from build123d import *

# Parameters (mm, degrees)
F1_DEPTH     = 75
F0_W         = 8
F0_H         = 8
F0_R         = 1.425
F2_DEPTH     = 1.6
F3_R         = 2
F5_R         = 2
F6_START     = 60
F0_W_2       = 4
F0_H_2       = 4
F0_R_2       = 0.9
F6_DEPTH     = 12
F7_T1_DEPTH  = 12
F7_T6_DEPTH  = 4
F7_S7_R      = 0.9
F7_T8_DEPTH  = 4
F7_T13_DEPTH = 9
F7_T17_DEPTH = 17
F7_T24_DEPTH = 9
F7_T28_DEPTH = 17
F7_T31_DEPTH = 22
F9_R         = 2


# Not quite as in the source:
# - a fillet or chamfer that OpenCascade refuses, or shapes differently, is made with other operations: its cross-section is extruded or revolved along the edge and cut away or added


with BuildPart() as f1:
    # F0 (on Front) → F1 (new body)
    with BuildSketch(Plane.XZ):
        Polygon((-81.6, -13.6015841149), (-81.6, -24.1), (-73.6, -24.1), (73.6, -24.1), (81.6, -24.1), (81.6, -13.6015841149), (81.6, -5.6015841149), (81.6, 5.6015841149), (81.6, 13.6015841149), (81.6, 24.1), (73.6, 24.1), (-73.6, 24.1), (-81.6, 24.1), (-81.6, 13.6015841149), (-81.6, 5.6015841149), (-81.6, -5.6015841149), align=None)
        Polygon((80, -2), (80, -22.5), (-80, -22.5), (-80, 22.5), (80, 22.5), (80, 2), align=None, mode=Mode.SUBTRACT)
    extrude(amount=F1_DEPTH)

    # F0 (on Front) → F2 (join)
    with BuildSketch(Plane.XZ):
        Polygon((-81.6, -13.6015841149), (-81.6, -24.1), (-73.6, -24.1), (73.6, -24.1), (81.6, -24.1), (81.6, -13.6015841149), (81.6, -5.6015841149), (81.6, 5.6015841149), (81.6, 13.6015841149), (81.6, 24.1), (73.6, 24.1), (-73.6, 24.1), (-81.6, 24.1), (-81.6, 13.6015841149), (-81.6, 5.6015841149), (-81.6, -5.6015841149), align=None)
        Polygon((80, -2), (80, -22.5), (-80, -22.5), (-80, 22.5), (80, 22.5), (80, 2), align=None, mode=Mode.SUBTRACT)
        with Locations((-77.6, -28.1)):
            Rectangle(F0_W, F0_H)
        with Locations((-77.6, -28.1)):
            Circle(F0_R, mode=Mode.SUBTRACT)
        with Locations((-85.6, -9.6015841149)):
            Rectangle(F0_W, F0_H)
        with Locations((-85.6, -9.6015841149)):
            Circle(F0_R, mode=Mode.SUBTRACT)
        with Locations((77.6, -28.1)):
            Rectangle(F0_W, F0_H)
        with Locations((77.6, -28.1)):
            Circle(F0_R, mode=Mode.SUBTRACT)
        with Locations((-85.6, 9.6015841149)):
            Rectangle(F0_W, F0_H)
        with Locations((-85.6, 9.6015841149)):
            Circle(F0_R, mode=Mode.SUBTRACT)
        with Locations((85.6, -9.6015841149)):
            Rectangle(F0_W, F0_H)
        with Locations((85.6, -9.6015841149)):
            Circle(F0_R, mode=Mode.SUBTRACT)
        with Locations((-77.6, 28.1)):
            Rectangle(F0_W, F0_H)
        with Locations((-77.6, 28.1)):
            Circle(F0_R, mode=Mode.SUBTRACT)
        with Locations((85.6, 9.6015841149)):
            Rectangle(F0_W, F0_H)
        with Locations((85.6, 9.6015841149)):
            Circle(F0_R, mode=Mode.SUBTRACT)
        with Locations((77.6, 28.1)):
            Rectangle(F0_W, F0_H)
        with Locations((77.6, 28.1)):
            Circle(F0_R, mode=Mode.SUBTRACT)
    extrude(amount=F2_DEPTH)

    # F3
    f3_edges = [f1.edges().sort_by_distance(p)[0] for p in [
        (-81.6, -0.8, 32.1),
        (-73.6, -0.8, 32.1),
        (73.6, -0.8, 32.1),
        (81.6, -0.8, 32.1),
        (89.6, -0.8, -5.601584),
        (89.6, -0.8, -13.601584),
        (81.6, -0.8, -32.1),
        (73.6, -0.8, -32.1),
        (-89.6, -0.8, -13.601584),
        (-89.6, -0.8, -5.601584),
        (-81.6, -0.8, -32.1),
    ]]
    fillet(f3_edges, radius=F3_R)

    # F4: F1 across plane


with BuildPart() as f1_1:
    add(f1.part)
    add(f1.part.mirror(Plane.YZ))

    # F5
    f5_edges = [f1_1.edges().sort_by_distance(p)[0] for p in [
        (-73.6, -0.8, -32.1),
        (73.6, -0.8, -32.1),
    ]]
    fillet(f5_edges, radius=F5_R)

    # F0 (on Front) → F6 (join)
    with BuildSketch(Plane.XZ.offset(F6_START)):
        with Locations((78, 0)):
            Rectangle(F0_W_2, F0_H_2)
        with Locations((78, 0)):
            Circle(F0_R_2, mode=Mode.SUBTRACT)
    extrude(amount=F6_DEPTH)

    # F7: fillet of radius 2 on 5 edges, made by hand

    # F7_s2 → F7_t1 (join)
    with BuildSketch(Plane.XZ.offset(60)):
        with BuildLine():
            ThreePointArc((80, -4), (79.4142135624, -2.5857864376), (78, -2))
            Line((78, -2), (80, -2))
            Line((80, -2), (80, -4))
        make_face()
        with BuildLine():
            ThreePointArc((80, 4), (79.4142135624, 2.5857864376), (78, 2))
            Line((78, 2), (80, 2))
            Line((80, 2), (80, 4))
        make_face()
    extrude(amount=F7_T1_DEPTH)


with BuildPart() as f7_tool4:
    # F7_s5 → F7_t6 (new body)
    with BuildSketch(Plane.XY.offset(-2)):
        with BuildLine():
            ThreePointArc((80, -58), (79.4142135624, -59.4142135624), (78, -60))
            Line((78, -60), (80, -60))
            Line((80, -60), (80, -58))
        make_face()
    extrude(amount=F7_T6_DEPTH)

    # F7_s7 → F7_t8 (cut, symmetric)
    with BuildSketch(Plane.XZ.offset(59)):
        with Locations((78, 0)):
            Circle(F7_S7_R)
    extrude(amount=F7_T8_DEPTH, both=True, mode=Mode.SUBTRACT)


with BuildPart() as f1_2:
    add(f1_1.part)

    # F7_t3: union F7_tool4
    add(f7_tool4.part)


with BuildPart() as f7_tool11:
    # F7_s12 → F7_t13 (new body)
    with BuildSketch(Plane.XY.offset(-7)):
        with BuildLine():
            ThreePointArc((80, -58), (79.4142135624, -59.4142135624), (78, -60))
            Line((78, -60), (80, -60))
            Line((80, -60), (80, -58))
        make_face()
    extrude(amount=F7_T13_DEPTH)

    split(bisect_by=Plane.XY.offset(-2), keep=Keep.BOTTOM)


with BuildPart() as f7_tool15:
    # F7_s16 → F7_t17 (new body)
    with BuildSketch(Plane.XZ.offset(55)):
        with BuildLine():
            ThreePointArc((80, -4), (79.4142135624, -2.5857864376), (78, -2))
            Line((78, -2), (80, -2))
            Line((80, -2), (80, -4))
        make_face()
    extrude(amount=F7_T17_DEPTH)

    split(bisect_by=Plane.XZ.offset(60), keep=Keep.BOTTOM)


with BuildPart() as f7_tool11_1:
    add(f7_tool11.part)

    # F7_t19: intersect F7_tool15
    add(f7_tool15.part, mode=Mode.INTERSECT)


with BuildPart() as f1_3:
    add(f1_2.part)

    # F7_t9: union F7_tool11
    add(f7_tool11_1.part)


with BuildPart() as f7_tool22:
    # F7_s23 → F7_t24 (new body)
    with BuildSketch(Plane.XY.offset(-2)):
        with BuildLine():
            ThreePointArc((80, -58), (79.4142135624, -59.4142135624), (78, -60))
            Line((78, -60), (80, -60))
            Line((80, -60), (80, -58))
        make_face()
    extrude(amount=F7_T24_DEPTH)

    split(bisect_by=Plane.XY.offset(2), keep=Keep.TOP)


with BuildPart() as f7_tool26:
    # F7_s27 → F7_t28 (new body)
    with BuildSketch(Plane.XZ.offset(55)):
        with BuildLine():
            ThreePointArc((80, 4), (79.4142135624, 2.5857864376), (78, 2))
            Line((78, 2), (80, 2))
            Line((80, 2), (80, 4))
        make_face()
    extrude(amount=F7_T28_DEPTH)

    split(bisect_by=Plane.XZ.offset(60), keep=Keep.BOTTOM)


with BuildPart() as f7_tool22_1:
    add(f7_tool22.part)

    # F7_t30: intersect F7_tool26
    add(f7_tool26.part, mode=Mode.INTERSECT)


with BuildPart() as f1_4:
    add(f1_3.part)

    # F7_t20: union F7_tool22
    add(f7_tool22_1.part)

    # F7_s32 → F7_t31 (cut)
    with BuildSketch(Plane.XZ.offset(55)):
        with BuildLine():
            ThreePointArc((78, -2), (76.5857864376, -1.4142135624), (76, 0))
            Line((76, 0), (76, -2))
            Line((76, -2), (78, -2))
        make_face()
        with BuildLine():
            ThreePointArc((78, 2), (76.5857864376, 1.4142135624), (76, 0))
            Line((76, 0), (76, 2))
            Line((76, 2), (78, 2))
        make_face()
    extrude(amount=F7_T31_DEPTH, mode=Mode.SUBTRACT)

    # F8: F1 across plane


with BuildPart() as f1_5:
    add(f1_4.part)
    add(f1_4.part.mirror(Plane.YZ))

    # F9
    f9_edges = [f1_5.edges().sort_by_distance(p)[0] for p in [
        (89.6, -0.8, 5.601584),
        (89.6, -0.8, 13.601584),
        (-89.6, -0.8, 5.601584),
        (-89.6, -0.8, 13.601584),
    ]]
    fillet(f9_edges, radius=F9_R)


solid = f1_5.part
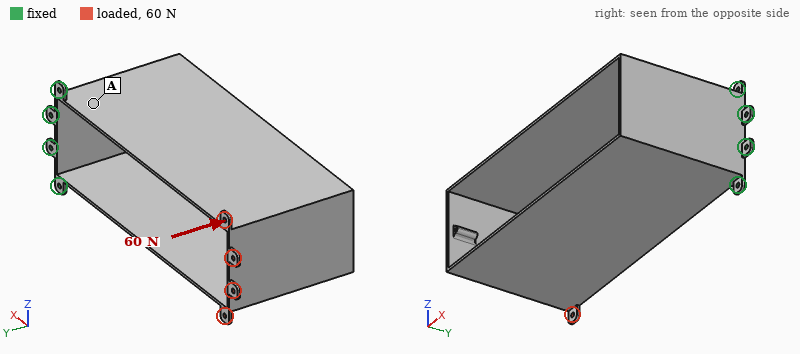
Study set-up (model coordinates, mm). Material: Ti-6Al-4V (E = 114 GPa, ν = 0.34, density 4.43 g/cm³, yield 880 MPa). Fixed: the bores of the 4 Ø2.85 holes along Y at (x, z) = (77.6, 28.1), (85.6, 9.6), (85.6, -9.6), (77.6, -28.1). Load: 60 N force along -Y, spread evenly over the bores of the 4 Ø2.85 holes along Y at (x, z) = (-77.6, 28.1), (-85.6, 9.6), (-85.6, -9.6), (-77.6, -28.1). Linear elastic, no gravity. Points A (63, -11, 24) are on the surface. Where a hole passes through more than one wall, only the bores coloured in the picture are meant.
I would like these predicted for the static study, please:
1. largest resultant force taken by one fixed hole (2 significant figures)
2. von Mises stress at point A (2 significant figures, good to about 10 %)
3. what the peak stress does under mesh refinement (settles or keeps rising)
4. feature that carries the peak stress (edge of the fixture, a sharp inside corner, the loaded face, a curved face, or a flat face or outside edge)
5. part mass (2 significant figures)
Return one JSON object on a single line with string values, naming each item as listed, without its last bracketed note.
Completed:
{"largest resultant force taken by one fixed hole": "560 N", "von Mises stress at point A": "20 MPa", "what the peak stress does under mesh refinement": "keeps rising", "feature that carries the peak stress": "edge of the fixture", "part mass": "230 g"}
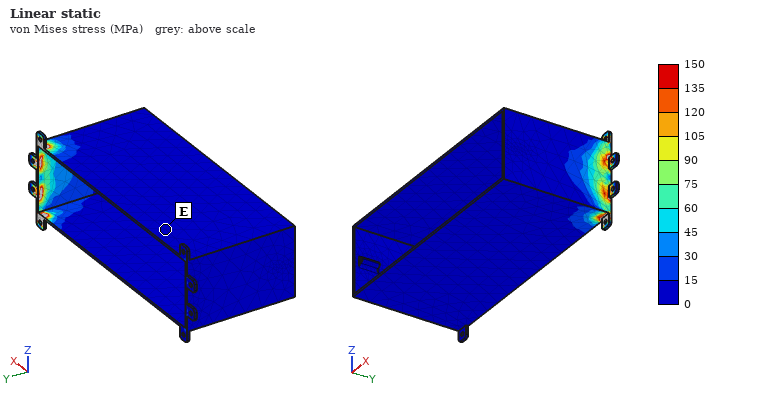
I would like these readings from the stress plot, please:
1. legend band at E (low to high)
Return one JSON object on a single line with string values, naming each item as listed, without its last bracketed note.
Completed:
{"legend band at E": "0 to 15 MPa"}
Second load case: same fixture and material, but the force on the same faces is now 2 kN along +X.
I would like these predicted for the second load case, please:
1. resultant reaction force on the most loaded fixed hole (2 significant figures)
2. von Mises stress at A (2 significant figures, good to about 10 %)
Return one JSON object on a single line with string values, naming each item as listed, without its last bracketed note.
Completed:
{"resultant reaction force on the most loaded fixed hole": "990 N", "von Mises stress at A": "42 MPa"}
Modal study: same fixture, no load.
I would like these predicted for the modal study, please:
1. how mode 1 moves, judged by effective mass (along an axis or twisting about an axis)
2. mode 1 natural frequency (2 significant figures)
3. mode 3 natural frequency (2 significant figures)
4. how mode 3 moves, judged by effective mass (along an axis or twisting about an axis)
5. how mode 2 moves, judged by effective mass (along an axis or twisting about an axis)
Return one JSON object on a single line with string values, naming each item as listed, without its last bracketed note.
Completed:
{"how mode 1 moves, judged by effective mass": "along Z", "mode 1 natural frequency": "61 Hz", "mode 3 natural frequency": "210 Hz", "how mode 3 moves, judged by effective mass": "twisting about X", "how mode 2 moves, judged by effective mass": "along Y"}
